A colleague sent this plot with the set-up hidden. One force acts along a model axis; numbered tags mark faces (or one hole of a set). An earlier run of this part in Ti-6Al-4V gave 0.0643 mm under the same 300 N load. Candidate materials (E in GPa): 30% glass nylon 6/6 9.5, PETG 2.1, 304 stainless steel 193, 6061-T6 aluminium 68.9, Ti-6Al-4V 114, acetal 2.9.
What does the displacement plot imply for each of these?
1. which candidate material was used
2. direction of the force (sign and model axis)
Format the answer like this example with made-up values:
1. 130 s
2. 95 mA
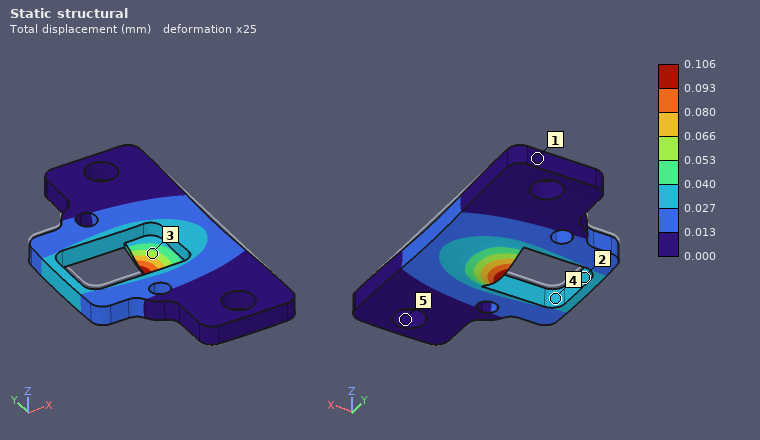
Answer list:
1. 6061-T6 aluminium
2. -Z
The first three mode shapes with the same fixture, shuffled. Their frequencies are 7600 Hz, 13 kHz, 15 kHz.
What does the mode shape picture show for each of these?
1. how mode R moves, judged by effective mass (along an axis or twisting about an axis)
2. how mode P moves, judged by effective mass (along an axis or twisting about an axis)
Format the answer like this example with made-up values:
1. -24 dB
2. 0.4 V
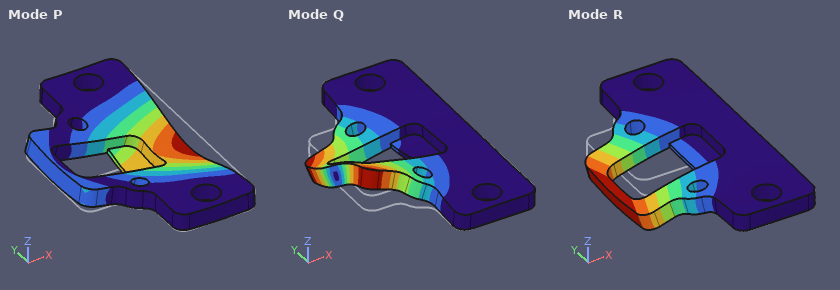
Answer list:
1. along Z
2. along Z
